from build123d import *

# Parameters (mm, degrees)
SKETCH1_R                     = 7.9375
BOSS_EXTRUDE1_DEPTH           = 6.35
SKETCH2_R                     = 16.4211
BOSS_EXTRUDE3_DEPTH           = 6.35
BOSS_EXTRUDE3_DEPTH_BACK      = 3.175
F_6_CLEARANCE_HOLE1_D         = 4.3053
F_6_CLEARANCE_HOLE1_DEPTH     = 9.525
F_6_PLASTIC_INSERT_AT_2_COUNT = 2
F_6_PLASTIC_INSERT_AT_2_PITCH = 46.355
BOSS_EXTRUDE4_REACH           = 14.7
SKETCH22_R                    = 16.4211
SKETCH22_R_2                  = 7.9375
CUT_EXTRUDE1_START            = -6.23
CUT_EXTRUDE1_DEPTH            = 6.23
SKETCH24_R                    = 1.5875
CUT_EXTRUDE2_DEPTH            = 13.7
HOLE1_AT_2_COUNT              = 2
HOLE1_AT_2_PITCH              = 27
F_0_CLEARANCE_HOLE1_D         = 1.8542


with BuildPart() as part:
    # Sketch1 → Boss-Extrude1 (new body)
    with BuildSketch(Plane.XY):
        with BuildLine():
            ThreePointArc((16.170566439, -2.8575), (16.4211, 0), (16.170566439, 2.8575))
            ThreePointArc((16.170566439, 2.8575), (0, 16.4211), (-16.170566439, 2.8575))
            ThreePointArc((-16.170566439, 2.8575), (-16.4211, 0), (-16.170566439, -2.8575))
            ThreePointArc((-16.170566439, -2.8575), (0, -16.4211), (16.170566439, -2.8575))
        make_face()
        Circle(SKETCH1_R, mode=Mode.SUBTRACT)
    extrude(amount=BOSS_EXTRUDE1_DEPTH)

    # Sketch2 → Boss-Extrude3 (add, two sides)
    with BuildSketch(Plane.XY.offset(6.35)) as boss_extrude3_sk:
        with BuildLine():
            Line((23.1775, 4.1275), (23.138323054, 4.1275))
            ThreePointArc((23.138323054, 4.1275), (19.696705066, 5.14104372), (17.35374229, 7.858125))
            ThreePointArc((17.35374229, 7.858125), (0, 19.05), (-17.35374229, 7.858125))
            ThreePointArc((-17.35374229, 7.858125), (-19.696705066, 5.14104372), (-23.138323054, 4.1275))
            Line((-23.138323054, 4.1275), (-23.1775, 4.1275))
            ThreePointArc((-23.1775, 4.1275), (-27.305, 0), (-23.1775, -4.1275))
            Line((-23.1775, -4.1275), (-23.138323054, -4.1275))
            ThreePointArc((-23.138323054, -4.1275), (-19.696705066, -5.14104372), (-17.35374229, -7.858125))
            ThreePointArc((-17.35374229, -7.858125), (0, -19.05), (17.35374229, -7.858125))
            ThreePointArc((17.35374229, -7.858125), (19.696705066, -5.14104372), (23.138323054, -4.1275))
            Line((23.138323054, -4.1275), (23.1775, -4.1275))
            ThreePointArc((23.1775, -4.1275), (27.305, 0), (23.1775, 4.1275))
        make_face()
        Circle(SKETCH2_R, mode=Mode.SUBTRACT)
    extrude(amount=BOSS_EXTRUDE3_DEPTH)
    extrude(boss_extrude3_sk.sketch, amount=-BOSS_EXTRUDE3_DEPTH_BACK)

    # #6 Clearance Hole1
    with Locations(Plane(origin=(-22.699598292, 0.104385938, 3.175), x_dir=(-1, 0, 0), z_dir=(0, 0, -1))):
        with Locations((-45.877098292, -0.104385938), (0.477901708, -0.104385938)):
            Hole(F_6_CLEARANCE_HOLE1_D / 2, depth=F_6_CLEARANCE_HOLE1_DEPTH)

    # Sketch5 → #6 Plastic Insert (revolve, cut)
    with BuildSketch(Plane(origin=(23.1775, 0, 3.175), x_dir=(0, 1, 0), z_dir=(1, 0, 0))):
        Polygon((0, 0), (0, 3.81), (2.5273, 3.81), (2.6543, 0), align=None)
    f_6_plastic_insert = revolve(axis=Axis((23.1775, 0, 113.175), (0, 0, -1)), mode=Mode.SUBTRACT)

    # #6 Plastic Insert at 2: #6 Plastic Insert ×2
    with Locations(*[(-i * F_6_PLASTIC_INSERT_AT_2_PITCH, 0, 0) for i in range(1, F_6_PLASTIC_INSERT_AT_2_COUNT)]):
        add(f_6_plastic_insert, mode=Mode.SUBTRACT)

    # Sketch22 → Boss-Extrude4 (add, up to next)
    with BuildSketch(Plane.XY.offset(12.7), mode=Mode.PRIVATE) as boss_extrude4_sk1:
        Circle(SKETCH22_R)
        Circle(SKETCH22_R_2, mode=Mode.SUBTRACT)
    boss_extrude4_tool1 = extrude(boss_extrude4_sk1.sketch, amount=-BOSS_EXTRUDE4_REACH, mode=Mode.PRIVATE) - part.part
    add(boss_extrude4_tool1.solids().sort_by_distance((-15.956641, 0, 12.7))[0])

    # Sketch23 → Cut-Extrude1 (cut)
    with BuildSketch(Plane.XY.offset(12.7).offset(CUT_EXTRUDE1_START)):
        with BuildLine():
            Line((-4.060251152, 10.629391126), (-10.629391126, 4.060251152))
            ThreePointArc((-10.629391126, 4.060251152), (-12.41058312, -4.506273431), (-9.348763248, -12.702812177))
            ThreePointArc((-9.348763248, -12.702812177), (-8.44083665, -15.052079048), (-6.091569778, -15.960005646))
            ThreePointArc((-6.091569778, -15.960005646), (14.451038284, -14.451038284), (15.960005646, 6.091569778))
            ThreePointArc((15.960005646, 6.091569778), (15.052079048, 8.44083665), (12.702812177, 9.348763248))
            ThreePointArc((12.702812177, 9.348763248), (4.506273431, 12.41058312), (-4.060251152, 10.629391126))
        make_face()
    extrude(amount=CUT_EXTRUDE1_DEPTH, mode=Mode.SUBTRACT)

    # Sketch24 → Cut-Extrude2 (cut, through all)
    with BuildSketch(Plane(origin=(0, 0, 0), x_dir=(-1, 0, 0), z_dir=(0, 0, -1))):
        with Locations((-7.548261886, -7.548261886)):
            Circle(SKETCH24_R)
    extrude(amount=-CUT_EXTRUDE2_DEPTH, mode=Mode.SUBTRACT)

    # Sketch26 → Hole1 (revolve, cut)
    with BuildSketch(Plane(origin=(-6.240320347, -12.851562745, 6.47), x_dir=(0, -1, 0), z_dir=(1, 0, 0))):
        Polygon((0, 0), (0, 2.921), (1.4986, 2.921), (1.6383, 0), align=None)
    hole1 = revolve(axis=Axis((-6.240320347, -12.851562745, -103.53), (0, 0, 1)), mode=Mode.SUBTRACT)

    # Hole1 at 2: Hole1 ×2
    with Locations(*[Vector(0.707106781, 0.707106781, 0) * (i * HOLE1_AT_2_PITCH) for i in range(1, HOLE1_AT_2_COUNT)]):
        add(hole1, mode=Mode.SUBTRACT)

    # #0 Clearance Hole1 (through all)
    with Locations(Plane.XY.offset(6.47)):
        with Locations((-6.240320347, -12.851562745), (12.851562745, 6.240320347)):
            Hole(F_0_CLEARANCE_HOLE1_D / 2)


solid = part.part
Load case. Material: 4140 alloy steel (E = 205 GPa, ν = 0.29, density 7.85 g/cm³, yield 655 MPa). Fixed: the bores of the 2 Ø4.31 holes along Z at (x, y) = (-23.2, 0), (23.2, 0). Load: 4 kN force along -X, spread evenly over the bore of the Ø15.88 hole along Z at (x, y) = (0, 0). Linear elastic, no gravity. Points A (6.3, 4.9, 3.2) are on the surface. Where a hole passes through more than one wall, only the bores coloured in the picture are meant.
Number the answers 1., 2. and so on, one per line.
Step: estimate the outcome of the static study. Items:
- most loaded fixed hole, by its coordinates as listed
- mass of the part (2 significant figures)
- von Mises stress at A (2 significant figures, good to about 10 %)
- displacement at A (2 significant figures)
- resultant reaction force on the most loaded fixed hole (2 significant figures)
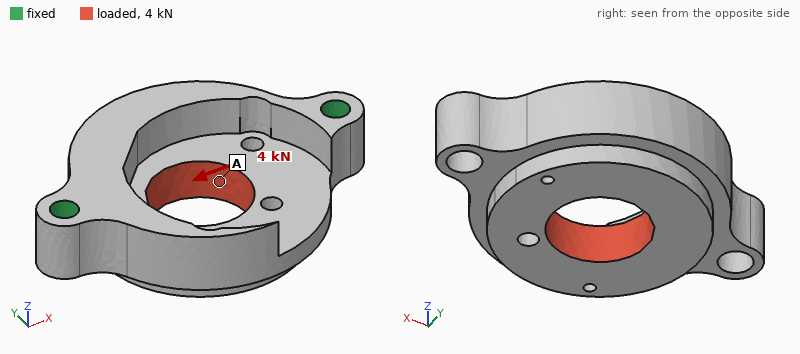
1. (-23.2, 0)
2. 66 g
3. 21 MPa
4. 3.9 µm
5. 2.3 kN
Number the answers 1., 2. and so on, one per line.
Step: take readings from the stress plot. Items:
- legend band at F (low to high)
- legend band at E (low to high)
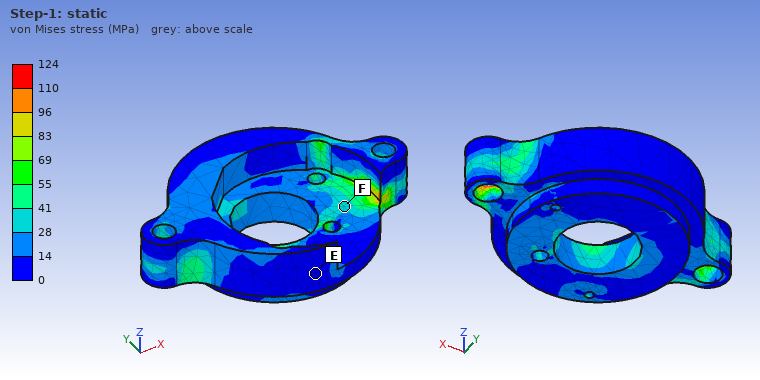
1. 28 to 41 MPa
2. 0 to 14 MPa
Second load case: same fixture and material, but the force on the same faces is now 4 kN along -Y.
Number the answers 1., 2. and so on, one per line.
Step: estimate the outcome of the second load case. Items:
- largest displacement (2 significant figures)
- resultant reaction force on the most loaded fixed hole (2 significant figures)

1. 33 µm
2. 2.0 kN
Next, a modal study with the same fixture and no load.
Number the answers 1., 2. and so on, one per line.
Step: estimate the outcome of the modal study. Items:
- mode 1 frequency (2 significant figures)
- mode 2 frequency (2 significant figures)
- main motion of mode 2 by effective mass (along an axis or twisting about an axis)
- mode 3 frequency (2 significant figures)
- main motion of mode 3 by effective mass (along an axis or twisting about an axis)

1. 6900 Hz
2. 11 kHz
3. along Z
4. 18 kHz
5. along Y
